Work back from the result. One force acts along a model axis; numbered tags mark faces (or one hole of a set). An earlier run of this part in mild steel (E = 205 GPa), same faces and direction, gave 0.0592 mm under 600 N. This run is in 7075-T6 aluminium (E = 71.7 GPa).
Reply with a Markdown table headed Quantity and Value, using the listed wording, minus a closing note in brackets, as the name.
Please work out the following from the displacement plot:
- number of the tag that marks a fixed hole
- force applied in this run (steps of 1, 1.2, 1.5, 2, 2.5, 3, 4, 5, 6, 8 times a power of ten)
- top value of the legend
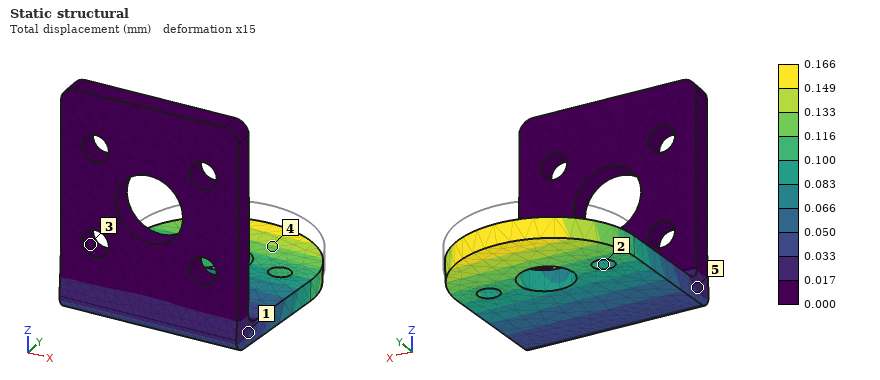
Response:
| Quantity | Value |
|---|---|
| number of the tag that marks a fixed hole | 3 |
| force applied in this run | 600 N |
| top value of the legend | 0.166 mm |
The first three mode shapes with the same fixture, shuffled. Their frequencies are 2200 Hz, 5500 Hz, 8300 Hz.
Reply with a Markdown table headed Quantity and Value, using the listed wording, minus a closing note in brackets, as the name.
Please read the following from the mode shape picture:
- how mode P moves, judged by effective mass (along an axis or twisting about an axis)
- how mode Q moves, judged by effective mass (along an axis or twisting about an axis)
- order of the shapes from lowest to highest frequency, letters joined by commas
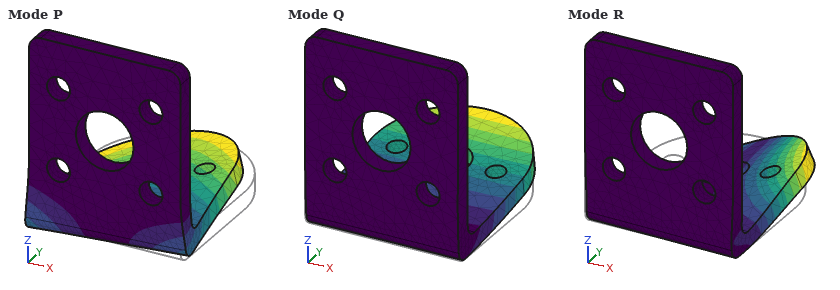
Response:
| Quantity | Value |
|---|---|
| how mode P moves, judged by effective mass | along X |
| how mode Q moves, judged by effective mass | along Z |
| order of the shapes from lowest to highest frequency, letters joined by commas | Q, P, R |
